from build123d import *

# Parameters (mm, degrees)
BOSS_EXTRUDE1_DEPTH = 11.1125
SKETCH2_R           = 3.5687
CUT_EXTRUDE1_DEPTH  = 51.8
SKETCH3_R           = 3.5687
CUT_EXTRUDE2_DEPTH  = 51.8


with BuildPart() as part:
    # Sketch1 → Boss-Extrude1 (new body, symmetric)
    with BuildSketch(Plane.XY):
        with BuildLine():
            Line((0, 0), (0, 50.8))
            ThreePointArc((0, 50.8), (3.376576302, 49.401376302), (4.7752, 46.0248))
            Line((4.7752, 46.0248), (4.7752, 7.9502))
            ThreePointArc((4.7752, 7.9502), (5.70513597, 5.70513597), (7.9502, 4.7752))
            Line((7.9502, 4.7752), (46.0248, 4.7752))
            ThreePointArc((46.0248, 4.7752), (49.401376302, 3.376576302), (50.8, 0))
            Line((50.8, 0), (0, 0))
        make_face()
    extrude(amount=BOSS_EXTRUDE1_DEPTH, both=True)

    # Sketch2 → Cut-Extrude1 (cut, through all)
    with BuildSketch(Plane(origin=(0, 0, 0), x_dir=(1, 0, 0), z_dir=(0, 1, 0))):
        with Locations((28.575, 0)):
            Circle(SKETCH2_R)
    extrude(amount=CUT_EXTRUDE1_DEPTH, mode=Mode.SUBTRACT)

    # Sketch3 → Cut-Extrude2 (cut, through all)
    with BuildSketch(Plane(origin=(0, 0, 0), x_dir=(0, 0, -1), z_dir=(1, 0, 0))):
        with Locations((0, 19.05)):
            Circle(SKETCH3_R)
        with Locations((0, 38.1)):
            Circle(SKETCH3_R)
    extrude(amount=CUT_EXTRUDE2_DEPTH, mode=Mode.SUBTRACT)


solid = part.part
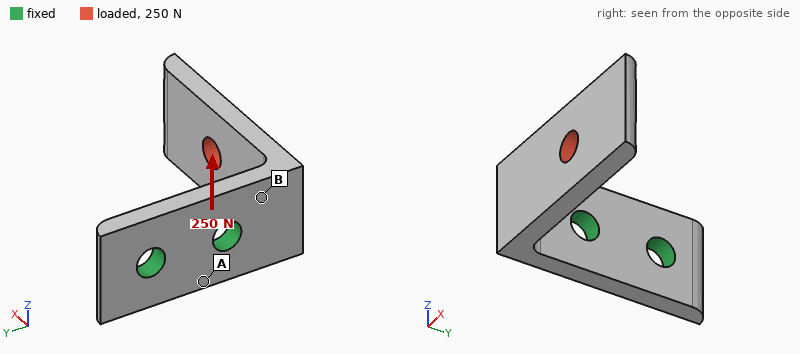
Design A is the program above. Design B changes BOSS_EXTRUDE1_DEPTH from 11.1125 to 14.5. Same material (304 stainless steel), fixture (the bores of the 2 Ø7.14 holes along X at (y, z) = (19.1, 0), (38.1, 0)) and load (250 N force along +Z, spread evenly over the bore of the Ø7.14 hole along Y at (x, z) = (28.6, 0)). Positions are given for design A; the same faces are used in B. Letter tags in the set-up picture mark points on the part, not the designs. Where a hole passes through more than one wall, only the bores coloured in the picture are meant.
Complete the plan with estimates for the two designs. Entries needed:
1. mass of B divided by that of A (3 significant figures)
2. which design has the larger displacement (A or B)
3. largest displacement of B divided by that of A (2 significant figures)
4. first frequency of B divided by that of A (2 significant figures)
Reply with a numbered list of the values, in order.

1. 1.32
2. A
3. 0.76
4. 0.99
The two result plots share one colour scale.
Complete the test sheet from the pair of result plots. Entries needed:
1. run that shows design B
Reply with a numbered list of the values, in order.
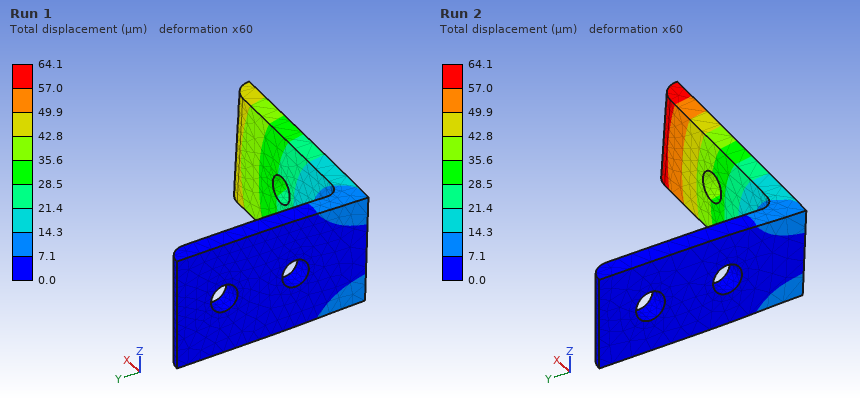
1. Run 1
